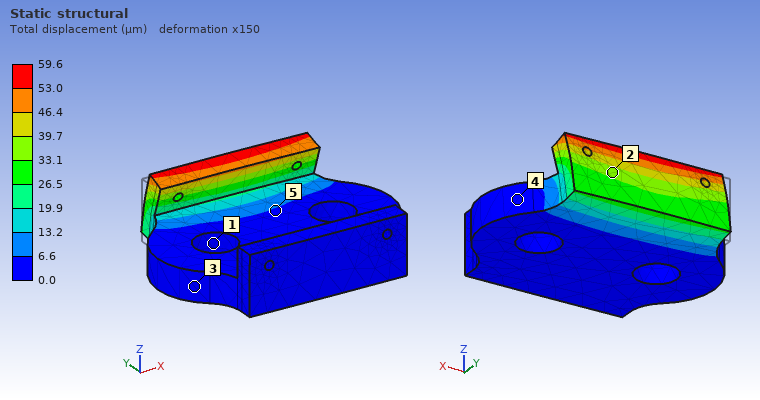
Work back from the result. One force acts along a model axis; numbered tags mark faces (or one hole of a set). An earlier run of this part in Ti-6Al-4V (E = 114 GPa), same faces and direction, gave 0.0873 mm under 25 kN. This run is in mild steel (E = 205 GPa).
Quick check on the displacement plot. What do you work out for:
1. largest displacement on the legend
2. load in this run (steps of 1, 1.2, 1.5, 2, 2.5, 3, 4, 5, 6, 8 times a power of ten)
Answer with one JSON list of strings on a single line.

["59.6 µm", "30 kN"]
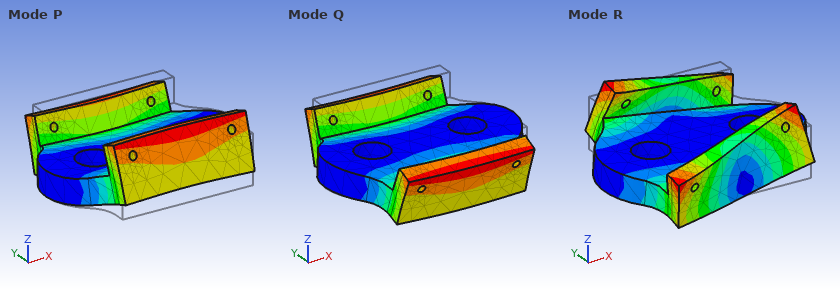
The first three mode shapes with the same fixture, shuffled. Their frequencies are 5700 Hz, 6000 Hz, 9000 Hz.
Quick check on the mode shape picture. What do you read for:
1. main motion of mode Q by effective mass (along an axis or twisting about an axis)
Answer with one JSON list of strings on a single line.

["along Z"]
